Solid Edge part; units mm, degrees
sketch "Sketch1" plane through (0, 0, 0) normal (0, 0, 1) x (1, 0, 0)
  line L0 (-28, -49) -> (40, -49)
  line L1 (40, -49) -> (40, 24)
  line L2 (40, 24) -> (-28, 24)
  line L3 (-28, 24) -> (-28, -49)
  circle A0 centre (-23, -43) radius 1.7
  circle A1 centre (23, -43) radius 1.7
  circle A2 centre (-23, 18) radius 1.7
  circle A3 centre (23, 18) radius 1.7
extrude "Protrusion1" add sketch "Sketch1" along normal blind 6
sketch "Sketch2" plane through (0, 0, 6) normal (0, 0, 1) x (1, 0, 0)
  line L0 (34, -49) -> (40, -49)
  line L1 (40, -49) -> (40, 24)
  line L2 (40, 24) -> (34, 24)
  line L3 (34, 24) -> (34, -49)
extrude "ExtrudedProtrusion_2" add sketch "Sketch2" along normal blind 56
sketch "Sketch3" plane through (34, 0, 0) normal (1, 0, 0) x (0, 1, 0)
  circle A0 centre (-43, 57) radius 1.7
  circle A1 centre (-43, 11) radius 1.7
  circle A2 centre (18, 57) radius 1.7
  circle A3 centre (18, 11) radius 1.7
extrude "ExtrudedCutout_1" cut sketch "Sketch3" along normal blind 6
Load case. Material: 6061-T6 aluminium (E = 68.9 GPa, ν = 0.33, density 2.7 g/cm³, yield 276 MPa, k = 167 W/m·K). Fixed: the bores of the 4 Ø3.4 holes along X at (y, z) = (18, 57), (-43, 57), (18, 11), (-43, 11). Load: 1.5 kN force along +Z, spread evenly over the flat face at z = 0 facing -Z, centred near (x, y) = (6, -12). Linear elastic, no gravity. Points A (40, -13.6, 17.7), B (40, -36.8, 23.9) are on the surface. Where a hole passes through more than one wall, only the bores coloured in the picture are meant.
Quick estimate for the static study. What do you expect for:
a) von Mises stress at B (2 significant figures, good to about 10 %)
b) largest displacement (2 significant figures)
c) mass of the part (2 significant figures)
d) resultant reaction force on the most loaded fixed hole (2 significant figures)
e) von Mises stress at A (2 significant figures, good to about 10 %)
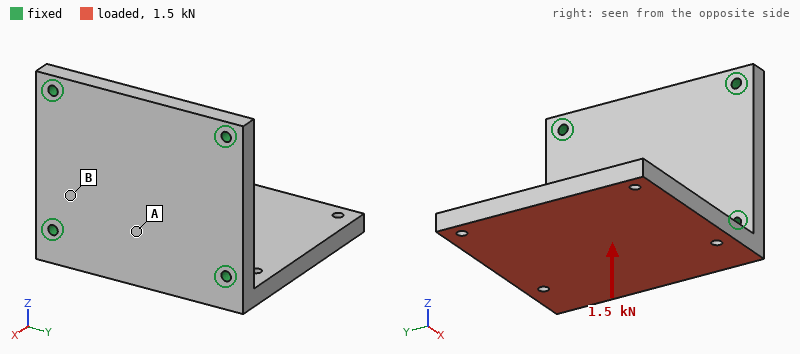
18 MPa
0.85 mm
150 g
530 N
42 MPa
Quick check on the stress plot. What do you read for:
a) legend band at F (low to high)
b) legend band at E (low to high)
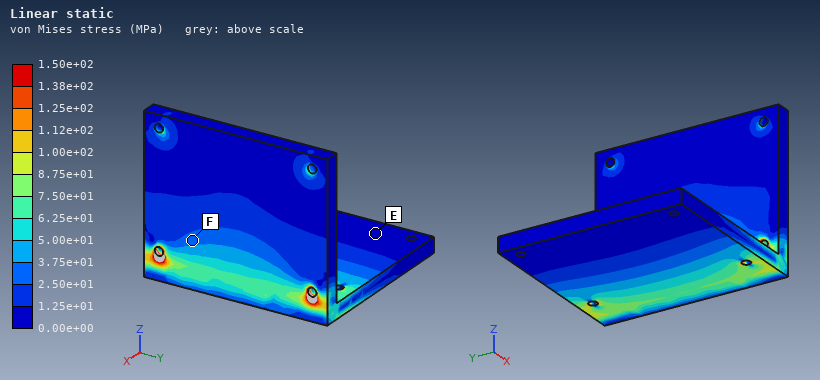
2.50e+01 to 3.75e+01 MPa
0.00e+00 to 1.25e+01 MPa
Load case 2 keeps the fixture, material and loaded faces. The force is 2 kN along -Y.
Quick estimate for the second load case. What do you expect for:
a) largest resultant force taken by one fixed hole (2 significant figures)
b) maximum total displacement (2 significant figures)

1.4 kN
36 µm
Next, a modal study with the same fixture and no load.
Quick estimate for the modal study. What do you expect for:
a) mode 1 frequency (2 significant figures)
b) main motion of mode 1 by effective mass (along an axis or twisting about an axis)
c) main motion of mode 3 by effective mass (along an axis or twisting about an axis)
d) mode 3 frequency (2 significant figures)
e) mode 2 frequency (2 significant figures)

930 Hz
along Z
along Y
5000 Hz
2400 Hz
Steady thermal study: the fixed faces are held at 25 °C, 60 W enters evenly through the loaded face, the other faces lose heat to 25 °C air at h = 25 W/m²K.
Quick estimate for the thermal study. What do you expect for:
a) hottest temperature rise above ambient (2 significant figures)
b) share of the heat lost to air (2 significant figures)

35 K
8.8 %
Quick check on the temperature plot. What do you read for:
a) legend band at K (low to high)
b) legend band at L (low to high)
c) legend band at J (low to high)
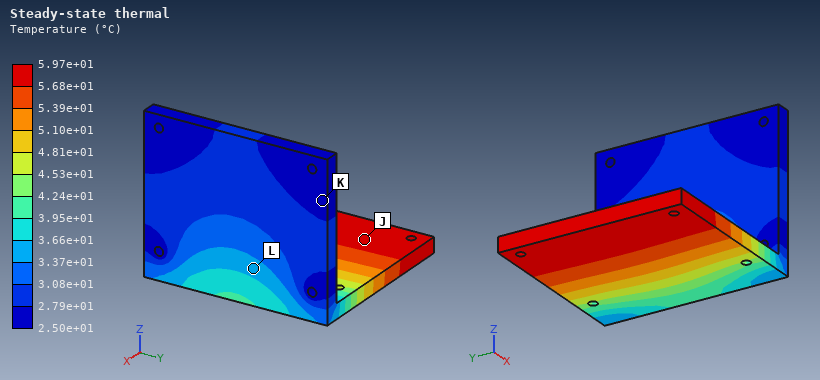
2.50e+01 to 2.79e+01 °C
3.37e+01 to 3.66e+01 °C
5.68e+01 to 5.97e+01 °C
